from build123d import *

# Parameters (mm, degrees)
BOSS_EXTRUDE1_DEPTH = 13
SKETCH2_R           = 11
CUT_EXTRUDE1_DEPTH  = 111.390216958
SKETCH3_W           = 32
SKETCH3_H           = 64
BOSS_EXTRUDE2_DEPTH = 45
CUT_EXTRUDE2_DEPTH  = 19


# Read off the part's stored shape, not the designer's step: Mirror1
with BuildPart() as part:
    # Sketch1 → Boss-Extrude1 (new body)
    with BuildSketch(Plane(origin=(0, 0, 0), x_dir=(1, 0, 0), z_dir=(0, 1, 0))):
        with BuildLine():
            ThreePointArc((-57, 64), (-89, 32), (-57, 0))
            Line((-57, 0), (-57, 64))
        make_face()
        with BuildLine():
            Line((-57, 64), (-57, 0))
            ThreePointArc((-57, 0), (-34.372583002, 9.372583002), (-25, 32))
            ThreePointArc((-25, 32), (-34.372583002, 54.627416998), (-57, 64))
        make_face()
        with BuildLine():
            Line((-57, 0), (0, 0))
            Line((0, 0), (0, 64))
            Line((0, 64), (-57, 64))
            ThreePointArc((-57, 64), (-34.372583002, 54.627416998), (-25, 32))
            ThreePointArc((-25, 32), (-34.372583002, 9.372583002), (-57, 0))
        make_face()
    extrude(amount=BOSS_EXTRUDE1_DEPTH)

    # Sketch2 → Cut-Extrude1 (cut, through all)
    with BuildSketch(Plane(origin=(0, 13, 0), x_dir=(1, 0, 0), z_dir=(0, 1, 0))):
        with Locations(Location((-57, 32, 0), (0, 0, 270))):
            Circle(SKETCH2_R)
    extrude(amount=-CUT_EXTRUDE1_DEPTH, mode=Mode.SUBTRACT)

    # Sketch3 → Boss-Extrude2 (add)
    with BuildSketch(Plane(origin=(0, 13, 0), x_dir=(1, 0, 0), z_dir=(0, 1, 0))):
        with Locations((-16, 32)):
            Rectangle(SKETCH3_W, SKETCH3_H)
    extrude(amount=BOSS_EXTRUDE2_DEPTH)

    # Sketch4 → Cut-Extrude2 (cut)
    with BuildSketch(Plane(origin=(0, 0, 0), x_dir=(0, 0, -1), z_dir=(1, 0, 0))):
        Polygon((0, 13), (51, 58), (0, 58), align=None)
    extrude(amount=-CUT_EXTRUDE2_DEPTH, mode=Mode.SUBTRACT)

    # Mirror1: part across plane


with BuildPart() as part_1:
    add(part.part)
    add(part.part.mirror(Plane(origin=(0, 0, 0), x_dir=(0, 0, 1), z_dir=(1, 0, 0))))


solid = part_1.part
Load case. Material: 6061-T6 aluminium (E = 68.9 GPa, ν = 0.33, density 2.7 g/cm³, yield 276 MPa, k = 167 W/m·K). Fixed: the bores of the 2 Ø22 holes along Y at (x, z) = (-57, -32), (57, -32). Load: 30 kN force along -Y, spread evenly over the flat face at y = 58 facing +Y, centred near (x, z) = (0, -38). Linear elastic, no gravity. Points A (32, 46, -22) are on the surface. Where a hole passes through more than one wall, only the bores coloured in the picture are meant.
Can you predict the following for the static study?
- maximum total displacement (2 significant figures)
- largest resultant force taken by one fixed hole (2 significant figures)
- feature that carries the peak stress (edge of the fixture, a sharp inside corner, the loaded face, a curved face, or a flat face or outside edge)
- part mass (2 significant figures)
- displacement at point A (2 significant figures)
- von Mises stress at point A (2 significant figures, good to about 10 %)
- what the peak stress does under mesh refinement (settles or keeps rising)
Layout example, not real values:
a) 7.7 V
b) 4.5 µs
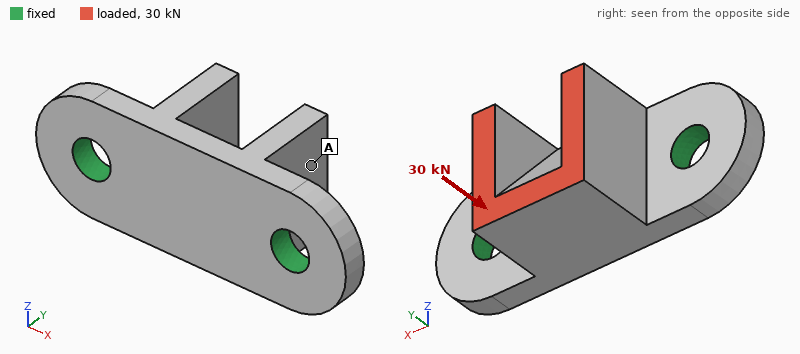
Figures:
a) 0.11 mm
b) 16 kN
c) edge of the fixture
d) 720 g
e) 0.062 mm
f) 17 MPa
g) keeps rising
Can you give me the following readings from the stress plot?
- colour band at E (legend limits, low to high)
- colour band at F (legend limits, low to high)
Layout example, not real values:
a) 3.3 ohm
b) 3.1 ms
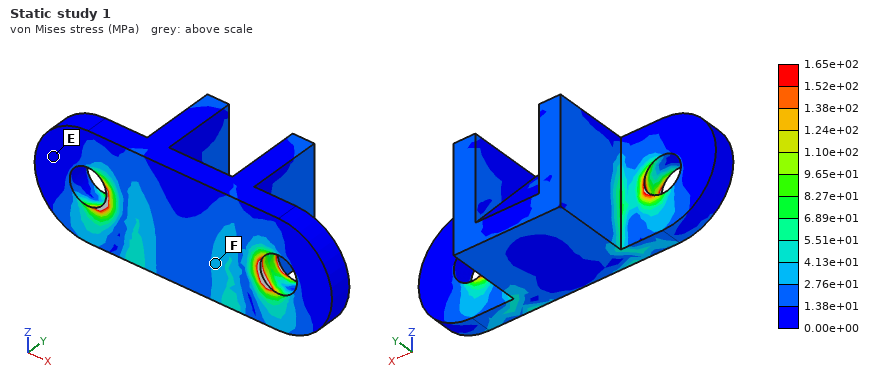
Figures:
a) 0.00e+00 to 1.38e+01 MPa
b) 2.76e+01 to 4.13e+01 MPa
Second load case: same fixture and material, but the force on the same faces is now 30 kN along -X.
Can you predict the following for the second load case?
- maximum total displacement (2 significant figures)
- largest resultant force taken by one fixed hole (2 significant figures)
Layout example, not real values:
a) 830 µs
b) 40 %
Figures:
a) 0.25 mm
b) 24 kN
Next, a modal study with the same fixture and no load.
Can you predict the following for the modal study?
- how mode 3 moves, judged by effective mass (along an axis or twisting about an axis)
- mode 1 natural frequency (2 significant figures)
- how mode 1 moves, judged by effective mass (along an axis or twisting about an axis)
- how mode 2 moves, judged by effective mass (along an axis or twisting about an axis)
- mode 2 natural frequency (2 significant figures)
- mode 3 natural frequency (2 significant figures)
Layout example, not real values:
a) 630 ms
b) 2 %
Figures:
a) along X
b) 2600 Hz
c) along Z
d) along Y
e) 5100 Hz
f) 6000 Hz
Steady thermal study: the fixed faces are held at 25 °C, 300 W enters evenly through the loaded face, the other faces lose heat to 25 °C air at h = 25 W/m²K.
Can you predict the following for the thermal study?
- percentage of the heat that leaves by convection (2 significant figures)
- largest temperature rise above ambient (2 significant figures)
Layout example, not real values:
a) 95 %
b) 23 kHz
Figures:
a) 7.5 %
b) 60 K
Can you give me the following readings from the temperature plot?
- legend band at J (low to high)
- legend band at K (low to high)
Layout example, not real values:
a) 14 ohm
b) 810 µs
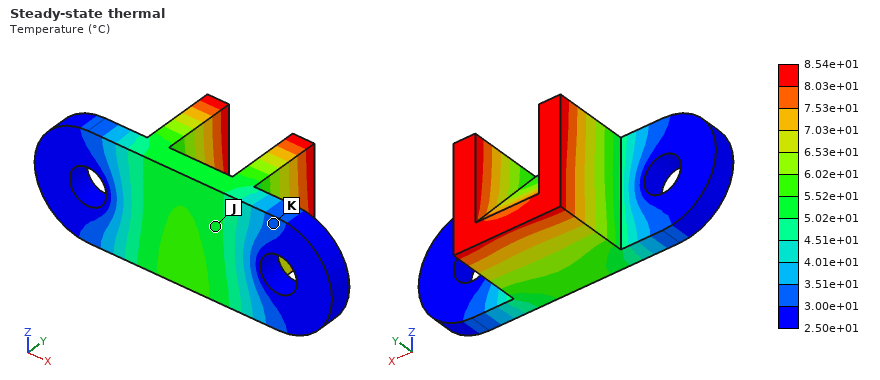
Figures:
a) 5.02e+01 to 5.52e+01 °C
b) 3.00e+01 to 3.51e+01 °C
